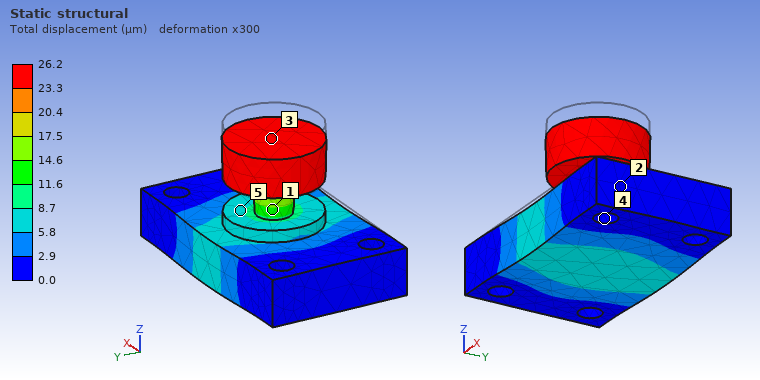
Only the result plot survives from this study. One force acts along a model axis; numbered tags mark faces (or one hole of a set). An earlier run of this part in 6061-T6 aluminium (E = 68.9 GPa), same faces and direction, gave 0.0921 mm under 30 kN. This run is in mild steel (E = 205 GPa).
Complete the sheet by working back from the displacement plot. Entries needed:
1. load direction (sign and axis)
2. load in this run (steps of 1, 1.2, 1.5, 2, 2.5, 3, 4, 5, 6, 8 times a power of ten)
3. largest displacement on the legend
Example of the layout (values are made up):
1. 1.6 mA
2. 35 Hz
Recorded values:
1. -Z
2. 25 kN
3. 26.2 µm
